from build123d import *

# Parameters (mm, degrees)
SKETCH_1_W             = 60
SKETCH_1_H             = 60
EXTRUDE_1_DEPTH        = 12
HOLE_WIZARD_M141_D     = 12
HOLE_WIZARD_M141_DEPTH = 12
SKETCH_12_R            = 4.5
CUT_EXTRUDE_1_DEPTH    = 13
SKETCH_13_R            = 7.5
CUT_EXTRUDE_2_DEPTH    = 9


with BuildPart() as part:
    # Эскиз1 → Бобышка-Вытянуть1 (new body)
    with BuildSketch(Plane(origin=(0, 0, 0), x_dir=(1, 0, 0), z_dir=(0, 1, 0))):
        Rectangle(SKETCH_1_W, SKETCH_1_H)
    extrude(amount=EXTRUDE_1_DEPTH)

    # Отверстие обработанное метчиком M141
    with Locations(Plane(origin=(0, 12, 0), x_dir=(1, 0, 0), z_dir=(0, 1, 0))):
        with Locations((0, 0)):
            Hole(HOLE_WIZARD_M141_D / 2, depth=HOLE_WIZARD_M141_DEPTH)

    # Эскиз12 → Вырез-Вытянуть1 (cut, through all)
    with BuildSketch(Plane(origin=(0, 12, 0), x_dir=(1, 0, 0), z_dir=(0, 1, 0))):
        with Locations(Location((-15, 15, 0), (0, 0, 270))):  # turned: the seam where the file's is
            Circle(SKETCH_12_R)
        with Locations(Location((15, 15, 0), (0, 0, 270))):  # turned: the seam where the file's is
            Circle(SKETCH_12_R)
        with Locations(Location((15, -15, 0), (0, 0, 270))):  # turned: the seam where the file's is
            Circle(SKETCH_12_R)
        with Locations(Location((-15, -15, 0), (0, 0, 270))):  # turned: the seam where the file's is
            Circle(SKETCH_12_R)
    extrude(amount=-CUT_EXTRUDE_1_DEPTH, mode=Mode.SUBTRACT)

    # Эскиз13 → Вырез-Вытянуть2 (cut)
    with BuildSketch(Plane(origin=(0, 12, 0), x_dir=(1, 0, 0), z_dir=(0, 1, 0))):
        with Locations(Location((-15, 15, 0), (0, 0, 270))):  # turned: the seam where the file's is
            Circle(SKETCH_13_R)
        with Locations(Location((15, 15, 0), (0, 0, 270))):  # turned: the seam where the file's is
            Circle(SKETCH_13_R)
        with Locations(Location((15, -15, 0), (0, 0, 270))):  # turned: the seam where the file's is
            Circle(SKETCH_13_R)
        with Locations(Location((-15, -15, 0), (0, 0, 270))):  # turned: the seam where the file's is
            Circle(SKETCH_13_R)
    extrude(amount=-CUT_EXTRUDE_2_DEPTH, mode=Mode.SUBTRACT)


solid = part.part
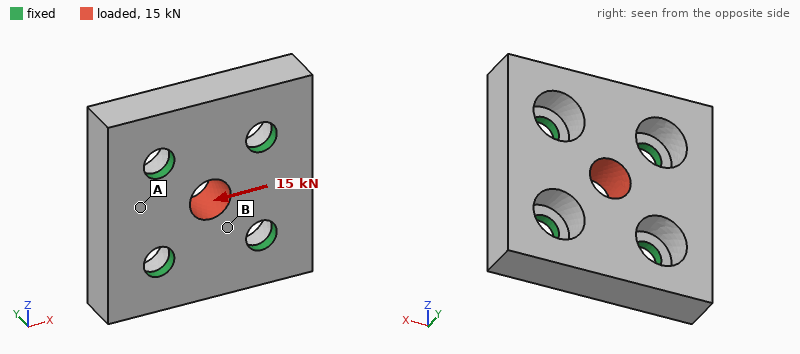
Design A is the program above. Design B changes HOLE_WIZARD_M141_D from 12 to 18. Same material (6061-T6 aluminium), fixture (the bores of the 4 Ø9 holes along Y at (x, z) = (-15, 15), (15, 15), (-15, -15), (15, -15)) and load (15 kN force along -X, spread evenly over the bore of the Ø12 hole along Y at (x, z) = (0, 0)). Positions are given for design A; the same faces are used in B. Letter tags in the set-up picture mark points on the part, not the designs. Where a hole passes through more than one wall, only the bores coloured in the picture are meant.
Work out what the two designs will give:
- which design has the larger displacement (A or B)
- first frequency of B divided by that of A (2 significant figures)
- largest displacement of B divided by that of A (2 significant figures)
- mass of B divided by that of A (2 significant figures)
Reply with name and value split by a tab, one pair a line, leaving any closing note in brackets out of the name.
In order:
which design has the larger displacement	B
first frequency of B divided by that of A	0.98
largest displacement of B divided by that of A	1.1
mass of B divided by that of A	0.95
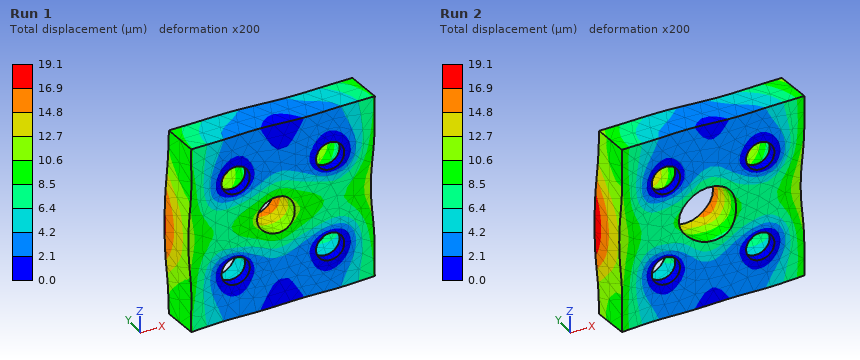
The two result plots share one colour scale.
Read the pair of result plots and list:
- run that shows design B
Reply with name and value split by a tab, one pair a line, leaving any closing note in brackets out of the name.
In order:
run that shows design B	Run 2
